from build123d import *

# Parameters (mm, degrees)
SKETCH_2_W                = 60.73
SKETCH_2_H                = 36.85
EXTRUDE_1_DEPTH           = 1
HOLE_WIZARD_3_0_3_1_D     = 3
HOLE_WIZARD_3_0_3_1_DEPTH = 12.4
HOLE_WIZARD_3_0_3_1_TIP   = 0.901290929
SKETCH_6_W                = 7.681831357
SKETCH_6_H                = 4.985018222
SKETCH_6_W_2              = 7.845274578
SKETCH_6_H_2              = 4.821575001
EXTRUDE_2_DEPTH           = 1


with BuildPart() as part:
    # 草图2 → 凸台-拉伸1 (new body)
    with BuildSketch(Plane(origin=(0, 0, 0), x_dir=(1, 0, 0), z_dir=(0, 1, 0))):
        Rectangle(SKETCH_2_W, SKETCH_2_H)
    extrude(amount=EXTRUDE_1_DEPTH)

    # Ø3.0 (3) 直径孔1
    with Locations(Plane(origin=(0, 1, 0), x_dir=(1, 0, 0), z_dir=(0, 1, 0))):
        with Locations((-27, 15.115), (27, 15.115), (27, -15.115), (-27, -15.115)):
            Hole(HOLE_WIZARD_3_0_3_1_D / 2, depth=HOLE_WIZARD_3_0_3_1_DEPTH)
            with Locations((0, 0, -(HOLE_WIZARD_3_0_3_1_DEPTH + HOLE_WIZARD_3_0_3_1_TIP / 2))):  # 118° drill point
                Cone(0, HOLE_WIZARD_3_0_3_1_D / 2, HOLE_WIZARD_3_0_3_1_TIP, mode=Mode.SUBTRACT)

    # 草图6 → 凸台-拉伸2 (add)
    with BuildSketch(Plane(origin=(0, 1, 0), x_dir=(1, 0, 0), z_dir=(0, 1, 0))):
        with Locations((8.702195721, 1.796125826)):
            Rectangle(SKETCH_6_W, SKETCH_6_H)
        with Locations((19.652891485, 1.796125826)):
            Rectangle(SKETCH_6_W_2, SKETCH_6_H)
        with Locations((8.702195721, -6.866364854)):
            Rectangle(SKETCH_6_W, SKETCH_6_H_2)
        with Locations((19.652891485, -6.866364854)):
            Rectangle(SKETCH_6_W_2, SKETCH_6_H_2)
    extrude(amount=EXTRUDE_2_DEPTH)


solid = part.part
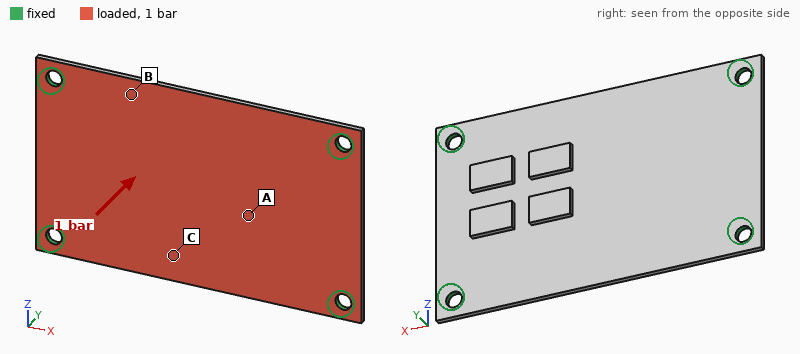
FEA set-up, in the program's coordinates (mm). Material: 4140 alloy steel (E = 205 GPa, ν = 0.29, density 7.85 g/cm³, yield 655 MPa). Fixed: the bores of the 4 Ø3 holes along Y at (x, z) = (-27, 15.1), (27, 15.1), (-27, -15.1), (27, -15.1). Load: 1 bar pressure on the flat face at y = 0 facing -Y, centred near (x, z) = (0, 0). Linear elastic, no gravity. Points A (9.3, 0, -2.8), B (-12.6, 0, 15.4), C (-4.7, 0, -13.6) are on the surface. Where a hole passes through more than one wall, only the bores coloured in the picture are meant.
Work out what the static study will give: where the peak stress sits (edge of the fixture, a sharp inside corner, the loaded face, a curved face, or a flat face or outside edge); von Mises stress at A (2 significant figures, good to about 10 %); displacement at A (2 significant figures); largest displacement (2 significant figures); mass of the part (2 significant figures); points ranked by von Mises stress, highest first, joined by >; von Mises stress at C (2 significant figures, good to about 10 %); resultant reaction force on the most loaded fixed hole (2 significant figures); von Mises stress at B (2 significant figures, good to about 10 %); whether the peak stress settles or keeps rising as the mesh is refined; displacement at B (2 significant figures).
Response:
edge of the fixture
21 MPa
0.11 mm
0.15 mm
19 g
C > B > A
73 MPa
57 N
38 MPa
keeps rising
0.086 mm
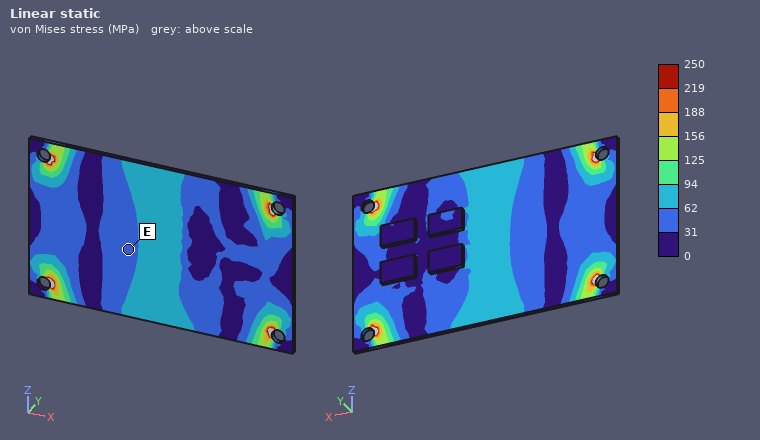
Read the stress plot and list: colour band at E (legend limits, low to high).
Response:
31 to 62 MPa
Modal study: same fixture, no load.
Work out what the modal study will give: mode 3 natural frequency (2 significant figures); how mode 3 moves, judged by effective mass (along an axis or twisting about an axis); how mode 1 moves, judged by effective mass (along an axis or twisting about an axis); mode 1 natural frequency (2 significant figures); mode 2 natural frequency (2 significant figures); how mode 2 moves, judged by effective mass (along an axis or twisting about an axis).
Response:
4400 Hz
twisting about Z
along Y
1700 Hz
2900 Hz
twisting about X
